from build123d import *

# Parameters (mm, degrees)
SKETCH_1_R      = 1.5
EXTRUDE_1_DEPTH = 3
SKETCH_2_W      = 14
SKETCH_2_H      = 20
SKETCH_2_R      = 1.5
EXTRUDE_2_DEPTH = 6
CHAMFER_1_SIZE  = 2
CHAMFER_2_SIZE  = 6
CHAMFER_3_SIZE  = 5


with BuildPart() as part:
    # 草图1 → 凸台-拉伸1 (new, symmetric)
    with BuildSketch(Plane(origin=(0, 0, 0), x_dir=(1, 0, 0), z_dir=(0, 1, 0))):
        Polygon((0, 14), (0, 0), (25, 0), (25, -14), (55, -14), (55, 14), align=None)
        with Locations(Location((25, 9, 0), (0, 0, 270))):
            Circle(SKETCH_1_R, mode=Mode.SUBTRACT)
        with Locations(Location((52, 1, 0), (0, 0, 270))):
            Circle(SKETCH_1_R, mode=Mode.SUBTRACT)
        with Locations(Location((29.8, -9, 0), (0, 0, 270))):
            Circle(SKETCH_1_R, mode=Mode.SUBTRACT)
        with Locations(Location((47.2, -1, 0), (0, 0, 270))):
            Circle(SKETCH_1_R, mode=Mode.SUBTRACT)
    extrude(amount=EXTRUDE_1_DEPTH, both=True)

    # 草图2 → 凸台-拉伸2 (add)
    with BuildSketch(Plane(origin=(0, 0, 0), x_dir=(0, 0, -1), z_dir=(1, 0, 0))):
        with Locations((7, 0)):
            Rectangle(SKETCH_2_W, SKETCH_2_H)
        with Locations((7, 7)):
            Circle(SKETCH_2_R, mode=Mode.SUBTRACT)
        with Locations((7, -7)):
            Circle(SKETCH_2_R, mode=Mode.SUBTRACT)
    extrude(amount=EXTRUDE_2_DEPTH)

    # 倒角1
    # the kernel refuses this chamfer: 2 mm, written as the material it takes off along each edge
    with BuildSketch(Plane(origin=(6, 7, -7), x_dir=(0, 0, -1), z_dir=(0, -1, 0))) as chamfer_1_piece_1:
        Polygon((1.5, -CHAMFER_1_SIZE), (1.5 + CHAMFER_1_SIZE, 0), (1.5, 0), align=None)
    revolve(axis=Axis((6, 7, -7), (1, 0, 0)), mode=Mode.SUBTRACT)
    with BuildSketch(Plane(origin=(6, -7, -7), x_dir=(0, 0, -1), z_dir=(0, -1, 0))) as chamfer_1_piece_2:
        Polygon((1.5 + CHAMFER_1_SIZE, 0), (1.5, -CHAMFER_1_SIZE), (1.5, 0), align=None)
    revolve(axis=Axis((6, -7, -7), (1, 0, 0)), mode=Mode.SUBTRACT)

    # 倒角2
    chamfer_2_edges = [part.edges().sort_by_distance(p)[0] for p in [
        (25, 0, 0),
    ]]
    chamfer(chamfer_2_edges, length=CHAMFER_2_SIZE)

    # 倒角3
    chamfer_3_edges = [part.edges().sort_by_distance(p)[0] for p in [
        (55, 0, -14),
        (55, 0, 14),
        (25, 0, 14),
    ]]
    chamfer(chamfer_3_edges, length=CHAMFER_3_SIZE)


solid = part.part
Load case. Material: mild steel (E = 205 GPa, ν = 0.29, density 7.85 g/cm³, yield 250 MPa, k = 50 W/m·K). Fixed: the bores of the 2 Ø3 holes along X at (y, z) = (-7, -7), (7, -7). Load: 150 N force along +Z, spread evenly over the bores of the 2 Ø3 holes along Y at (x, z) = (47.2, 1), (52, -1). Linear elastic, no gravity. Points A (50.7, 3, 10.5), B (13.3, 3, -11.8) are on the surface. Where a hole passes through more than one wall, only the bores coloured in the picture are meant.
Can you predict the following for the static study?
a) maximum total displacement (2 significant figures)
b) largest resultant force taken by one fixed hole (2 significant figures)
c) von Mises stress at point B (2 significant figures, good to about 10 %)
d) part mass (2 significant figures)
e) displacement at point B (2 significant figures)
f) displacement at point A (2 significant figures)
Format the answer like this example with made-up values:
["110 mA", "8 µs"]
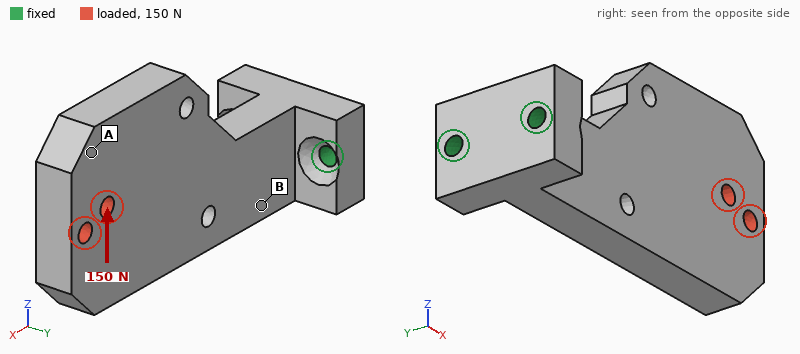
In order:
["47 µm", "75 N", "19 MPa", "62 g", "7.6 µm", "44 µm"]
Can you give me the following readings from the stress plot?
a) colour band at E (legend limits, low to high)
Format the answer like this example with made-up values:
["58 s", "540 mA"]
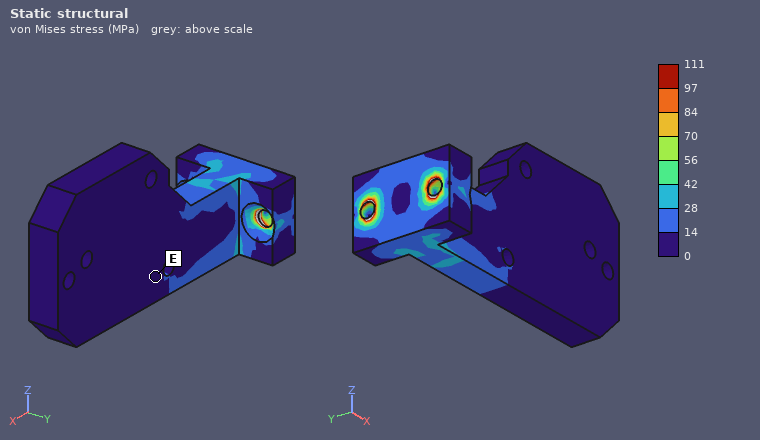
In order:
["0 to 14 MPa"]
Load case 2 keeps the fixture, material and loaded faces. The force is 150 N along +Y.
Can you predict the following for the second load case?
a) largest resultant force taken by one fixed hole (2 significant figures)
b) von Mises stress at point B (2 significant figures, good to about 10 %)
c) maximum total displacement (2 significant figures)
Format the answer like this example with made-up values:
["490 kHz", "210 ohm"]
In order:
["560 N", "63 MPa", "0.11 mm"]
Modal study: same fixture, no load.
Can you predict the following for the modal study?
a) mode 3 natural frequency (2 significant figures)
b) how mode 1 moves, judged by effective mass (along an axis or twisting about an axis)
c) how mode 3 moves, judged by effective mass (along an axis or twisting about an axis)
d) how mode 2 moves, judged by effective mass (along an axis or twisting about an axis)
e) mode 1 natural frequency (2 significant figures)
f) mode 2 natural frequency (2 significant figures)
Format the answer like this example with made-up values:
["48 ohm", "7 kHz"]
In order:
["4900 Hz", "along Y", "twisting about X", "along Z", "1400 Hz", "1900 Hz"]
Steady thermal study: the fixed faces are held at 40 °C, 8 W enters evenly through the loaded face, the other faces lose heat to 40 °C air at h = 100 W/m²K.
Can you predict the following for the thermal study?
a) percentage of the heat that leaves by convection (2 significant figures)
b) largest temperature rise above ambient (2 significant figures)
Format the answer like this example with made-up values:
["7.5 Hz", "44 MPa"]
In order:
["72 %", "35 K"]
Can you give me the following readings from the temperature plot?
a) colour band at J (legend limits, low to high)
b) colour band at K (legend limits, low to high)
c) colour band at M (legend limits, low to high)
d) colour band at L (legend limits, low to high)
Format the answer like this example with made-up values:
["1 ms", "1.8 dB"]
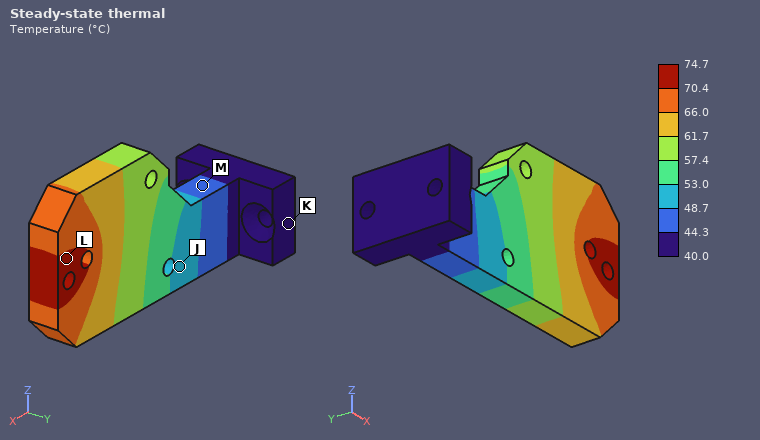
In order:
["48.7 to 53.0 °C", "40.0 to 44.3 °C", "44.3 to 48.7 °C", "70.4 to 74.7 °C"]
